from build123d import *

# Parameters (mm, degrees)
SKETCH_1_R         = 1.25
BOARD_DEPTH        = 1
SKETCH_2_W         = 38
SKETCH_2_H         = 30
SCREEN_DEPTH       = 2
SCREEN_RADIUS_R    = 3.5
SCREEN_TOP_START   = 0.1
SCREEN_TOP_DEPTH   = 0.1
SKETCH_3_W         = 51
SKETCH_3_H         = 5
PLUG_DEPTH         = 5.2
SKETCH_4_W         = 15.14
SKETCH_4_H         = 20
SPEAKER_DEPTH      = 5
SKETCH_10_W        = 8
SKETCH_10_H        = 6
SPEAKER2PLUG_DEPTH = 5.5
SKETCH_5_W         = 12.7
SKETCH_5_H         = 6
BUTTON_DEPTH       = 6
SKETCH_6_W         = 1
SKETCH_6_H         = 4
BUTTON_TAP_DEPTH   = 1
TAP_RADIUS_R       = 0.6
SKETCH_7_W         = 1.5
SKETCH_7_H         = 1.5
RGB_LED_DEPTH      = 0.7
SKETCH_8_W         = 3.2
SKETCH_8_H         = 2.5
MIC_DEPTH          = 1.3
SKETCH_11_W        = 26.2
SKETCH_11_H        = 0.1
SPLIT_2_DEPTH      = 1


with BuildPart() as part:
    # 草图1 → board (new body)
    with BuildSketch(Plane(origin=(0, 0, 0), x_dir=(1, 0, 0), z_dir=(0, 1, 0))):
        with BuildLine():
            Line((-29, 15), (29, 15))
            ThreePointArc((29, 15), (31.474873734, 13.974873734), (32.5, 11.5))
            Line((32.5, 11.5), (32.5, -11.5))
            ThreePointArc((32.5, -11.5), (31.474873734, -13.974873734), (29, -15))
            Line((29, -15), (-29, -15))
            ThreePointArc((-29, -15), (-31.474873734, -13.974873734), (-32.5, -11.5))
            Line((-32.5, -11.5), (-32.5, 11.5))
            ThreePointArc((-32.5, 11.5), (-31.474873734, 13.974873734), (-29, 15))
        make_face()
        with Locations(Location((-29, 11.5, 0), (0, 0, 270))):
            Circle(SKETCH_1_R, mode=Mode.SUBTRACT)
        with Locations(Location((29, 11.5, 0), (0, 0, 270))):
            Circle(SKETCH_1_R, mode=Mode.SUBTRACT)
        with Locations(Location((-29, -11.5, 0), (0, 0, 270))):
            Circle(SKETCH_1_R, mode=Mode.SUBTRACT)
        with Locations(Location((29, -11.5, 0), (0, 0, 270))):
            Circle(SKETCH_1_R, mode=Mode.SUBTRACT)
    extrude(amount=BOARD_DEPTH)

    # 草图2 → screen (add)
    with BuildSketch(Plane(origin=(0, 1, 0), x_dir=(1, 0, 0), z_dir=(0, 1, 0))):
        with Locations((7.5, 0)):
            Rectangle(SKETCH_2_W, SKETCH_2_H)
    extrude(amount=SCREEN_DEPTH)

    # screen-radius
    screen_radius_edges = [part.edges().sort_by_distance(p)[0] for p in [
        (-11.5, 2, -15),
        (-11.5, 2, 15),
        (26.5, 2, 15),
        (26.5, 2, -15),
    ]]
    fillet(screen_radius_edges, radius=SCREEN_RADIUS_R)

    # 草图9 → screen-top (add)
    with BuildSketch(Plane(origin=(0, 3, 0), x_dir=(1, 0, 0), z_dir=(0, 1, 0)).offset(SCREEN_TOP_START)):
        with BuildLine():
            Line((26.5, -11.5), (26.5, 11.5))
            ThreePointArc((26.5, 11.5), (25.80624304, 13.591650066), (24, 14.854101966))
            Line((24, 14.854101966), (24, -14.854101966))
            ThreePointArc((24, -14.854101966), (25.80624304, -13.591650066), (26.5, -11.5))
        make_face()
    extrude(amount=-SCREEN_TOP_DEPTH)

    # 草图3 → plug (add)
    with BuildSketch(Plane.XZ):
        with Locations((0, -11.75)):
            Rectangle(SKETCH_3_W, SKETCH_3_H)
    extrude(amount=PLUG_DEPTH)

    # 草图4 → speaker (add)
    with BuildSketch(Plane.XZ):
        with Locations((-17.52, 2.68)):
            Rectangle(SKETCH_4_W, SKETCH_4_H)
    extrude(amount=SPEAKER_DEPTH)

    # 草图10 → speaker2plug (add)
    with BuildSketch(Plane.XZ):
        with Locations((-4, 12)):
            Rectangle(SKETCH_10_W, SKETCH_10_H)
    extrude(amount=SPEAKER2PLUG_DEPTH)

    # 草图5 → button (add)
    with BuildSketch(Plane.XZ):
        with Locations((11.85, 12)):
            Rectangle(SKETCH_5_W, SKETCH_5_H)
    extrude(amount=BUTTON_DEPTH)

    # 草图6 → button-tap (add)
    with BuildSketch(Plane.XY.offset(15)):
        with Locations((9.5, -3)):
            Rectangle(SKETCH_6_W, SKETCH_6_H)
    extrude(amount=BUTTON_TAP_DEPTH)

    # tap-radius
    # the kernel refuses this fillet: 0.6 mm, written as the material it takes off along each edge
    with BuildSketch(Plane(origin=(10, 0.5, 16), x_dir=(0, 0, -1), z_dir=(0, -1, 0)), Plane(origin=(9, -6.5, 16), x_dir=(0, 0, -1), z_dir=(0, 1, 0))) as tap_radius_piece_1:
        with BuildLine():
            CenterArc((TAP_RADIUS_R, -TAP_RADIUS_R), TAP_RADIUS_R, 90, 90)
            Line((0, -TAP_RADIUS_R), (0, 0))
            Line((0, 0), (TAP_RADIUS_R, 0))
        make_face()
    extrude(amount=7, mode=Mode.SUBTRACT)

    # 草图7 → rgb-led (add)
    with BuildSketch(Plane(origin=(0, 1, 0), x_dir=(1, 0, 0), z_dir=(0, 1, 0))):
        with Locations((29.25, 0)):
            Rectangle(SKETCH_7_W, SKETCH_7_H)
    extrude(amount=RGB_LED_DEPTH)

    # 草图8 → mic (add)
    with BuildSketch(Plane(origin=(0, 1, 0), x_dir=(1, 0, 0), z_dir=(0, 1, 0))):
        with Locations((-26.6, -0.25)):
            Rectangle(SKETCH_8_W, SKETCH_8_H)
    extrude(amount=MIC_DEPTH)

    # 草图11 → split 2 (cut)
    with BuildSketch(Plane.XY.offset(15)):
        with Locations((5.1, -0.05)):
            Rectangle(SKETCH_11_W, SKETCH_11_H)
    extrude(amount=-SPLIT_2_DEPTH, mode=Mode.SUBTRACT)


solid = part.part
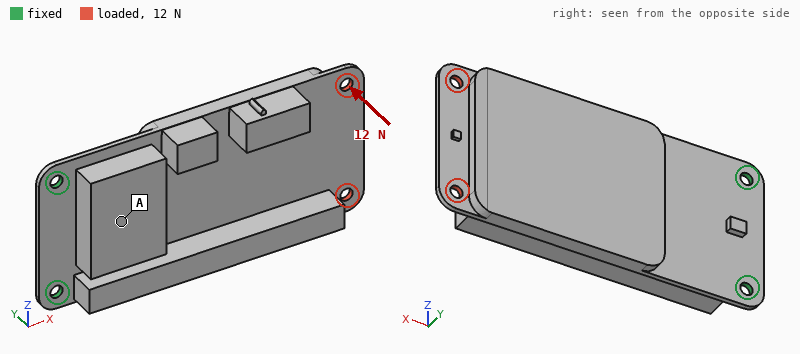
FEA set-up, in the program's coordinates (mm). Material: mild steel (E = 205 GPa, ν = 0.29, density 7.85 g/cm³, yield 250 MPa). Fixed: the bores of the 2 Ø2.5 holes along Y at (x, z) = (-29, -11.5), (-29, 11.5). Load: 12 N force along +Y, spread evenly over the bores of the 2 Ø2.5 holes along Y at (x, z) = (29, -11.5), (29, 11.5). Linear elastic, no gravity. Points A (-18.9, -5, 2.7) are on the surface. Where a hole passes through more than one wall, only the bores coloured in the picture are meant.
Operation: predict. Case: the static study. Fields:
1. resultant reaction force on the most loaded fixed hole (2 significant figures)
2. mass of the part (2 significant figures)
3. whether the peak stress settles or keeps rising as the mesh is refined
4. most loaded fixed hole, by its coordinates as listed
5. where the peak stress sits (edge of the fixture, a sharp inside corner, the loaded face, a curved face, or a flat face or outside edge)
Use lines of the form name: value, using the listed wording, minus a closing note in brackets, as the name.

resultant reaction force on the most loaded fixed hole: 10.0 N
mass of the part: 61 g
whether the peak stress settles or keeps rising as the mesh is refined: keeps rising
most loaded fixed hole, by its coordinates as listed: (-29, -11.5)
where the peak stress sits: edge of the fixture
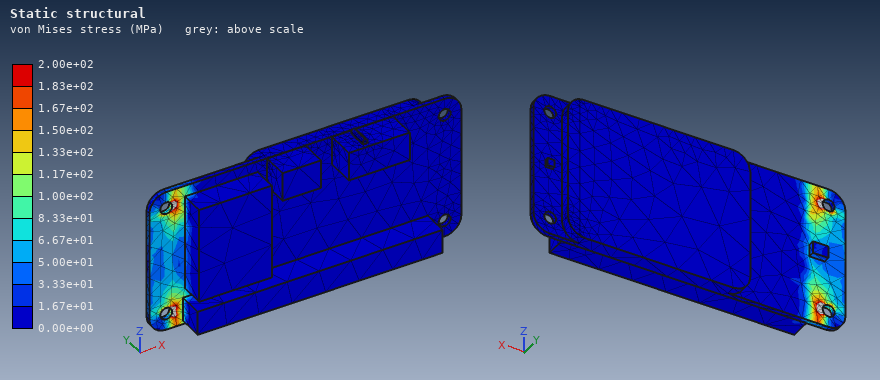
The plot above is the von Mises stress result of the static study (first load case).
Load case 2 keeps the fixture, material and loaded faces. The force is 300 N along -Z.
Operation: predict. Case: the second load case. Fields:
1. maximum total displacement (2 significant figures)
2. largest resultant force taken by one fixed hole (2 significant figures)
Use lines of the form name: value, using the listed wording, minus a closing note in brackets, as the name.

maximum total displacement: 39 µm
largest resultant force taken by one fixed hole: 760 N
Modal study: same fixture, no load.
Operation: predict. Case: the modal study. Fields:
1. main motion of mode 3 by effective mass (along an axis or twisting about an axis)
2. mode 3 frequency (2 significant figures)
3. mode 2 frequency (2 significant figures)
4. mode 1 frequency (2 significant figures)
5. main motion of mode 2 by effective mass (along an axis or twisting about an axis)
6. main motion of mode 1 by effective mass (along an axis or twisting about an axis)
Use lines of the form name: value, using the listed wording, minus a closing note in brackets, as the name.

main motion of mode 3 by effective mass: along Z
mode 3 frequency: 3700 Hz
mode 2 frequency: 2700 Hz
mode 1 frequency: 220 Hz
main motion of mode 2 by effective mass: twisting about X
main motion of mode 1 by effective mass: along Y
